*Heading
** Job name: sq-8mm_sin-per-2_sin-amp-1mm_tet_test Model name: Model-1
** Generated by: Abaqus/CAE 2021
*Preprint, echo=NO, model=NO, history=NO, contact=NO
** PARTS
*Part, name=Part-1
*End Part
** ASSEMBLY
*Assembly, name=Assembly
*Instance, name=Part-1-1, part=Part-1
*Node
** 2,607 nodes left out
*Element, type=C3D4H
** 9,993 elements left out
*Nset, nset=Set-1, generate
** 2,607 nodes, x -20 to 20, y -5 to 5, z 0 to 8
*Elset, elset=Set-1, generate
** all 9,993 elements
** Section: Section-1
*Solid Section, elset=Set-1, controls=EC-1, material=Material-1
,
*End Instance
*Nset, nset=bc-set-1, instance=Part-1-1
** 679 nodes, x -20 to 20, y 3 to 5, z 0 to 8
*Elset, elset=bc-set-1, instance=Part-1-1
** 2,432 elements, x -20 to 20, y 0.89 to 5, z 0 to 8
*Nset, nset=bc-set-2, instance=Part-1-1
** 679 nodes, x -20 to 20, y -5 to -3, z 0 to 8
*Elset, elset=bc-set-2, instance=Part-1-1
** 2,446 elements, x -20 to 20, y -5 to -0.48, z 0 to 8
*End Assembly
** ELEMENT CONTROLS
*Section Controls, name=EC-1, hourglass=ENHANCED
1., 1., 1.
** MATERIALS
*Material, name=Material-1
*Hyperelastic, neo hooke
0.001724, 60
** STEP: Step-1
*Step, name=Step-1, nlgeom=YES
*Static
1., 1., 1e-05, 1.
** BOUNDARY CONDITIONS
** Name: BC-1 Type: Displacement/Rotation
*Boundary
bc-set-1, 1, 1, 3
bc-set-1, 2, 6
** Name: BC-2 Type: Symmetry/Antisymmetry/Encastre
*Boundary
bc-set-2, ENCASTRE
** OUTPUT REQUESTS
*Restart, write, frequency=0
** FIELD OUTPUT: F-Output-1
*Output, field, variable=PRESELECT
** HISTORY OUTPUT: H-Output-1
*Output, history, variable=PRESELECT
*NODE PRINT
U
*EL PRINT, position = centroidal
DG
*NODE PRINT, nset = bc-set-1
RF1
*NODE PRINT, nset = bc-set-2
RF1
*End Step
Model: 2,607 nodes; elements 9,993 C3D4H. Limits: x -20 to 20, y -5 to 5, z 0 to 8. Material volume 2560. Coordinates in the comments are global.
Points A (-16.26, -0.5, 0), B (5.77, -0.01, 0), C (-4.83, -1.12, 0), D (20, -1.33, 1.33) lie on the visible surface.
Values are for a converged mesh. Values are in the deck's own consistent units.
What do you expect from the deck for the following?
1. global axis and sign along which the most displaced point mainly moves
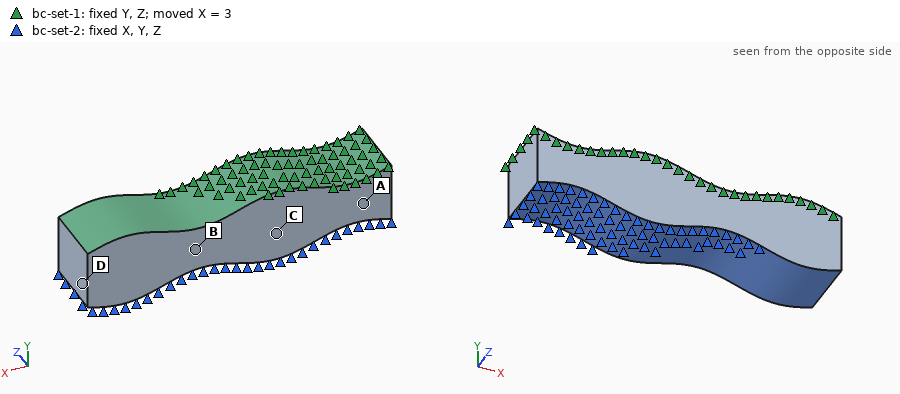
+X
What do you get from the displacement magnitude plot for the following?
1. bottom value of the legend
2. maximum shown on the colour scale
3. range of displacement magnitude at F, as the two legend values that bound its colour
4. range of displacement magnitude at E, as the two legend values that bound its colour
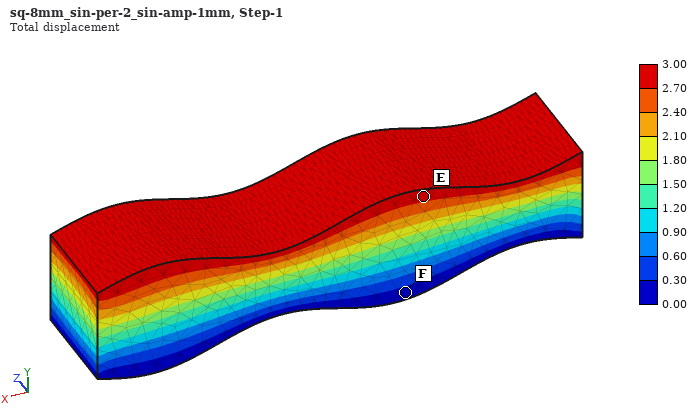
0.00
3.00
0.00 to 0.30
2.70 to 3.00
